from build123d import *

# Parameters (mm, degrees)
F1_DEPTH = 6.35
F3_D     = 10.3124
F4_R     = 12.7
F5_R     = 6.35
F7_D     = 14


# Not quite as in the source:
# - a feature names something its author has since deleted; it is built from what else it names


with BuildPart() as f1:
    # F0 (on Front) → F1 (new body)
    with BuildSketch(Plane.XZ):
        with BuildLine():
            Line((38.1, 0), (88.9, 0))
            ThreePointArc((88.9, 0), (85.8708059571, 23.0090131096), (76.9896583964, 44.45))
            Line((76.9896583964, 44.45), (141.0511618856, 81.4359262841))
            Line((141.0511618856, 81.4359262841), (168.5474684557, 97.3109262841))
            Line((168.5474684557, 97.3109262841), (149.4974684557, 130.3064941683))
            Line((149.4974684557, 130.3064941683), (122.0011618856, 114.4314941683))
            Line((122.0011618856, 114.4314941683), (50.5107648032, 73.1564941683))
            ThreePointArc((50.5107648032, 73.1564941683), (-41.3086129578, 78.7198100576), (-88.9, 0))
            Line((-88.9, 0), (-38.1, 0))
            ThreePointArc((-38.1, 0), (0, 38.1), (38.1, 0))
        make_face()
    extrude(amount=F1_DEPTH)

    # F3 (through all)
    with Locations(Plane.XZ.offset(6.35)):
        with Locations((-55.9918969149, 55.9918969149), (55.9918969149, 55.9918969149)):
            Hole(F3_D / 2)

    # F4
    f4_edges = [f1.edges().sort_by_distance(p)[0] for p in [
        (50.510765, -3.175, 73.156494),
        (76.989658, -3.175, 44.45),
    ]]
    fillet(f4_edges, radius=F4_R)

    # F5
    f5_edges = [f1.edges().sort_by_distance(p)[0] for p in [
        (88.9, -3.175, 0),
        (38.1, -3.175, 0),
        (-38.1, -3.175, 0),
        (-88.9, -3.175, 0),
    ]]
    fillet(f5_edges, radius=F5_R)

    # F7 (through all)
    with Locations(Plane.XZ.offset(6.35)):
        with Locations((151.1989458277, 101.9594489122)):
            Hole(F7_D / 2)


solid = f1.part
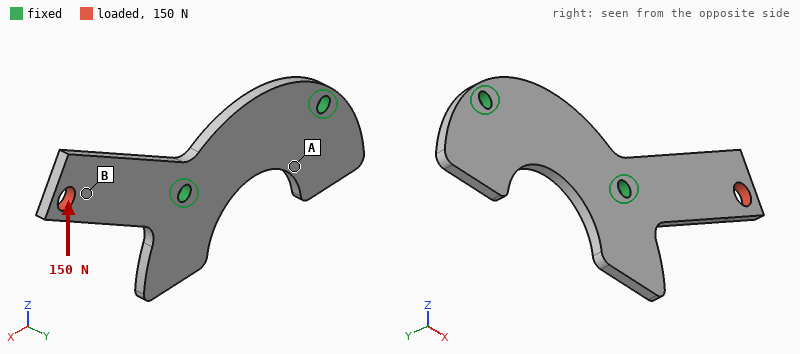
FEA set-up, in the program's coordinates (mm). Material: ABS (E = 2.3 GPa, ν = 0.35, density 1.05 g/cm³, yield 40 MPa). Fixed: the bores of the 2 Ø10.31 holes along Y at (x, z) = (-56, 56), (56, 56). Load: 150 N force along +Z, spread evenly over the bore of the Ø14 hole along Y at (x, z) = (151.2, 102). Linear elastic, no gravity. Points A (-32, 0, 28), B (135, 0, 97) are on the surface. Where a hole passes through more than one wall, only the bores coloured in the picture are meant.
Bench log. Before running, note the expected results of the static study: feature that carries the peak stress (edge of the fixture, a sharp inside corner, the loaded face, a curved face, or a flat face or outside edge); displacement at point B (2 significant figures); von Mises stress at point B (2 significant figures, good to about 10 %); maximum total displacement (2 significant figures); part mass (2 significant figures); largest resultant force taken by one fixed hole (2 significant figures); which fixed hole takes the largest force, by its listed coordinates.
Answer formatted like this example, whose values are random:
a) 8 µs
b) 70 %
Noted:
a) edge of the fixture
b) 0.78 mm
c) 1.9 MPa
d) 1.2 mm
e) 93 g
f) 240 N
g) (56, 56)
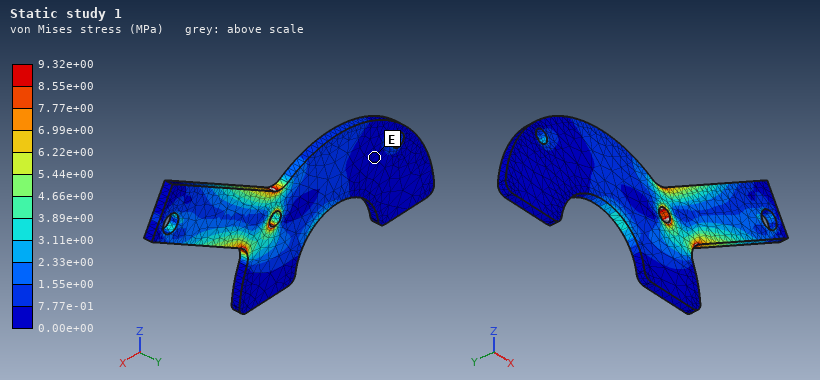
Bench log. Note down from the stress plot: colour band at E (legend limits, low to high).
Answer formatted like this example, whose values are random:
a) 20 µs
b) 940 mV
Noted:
a) 0.00e+00 to 7.77e-01 MPa
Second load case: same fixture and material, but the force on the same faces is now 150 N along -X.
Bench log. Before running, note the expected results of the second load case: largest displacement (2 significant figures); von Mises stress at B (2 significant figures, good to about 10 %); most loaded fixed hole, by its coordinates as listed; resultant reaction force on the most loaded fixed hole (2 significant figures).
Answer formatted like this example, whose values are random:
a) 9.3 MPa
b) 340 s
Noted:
a) 0.56 mm
b) 0.92 MPa
c) (56, 56)
d) 130 N
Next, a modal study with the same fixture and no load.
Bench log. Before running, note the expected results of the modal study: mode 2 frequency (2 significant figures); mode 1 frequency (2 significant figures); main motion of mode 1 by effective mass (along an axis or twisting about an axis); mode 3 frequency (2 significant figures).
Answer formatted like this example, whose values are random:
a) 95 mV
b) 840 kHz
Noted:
a) 490 Hz
b) 120 Hz
c) along Y
d) 520 Hz
